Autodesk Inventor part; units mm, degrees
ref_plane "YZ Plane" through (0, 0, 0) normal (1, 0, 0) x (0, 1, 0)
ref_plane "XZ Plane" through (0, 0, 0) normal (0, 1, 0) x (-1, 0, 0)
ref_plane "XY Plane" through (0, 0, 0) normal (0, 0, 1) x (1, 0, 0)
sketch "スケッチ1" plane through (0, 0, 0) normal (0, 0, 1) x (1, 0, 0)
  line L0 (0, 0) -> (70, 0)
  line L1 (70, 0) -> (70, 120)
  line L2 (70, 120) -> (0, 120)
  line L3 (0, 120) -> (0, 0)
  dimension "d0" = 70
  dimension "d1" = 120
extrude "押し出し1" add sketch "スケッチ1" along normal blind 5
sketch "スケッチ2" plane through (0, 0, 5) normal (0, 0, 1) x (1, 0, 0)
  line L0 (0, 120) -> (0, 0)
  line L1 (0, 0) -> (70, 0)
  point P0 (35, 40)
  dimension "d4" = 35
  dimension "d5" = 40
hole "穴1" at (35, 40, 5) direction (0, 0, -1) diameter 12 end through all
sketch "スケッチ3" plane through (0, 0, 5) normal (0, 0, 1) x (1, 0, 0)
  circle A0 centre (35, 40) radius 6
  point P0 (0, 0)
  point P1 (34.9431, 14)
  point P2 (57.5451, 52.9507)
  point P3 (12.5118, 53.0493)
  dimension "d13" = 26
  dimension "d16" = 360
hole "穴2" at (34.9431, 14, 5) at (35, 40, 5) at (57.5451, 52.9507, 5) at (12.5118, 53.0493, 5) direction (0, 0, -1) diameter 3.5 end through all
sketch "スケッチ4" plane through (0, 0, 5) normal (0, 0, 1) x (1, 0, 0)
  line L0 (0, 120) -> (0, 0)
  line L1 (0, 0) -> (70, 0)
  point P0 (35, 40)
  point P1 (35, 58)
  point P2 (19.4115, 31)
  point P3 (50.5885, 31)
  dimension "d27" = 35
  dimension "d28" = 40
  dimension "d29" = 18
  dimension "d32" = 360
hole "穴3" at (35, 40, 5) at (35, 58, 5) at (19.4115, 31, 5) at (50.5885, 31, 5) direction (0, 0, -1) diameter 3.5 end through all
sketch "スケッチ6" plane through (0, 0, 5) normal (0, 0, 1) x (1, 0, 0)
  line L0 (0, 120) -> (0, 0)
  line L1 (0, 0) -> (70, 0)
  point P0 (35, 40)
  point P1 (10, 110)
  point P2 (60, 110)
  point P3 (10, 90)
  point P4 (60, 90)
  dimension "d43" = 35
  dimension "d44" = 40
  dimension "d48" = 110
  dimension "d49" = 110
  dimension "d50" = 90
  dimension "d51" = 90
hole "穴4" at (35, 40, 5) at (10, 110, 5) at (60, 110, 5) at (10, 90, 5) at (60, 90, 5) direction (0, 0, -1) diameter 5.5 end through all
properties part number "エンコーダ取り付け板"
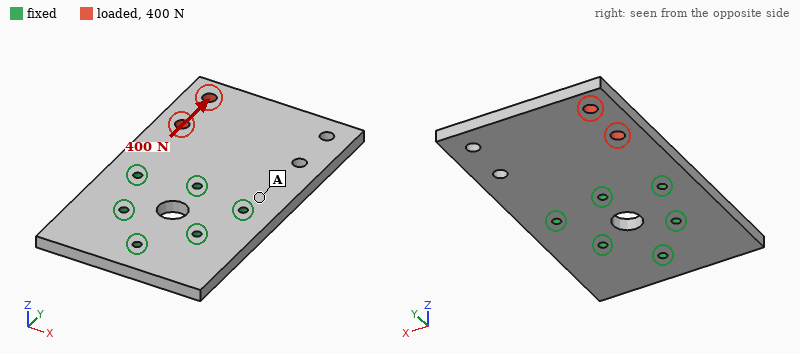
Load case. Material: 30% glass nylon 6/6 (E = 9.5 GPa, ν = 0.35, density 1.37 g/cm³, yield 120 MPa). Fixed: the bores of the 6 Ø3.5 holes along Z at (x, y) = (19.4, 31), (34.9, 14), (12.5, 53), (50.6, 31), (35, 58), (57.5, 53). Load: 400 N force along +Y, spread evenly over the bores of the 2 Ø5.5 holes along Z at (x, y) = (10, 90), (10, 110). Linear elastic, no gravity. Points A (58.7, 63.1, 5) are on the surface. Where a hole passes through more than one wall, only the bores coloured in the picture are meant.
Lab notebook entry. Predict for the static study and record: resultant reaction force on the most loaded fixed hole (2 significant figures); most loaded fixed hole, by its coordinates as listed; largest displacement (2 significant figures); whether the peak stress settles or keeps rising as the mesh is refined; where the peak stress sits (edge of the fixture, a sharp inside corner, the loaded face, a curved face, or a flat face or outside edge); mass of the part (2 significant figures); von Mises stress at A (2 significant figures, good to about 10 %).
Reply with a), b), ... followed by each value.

a) 280 N
b) (12.5, 53)
c) 29 µm
d) keeps rising
e) edge of the fixture
f) 56 g
g) 0.74 MPa
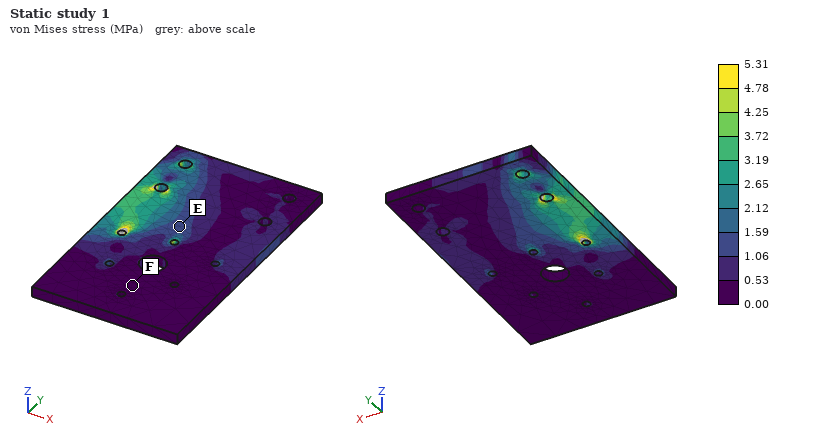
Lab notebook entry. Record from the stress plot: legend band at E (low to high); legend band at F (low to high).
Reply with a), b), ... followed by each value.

a) 1.06 to 1.59 MPa
b) 0.00 to 0.53 MPa
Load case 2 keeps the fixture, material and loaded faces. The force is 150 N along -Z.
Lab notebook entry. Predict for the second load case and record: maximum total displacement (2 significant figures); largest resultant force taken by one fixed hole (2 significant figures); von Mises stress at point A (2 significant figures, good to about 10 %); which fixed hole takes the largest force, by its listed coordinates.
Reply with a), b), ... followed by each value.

a) 1.5 mm
b) 180 N
c) 10 MPa
d) (35, 58)
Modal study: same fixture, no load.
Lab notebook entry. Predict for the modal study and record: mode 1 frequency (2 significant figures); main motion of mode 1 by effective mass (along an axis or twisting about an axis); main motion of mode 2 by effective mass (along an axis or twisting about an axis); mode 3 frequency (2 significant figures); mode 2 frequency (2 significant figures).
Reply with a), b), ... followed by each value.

a) 520 Hz
b) along Z
c) twisting about Y
d) 2800 Hz
e) 1100 Hz
